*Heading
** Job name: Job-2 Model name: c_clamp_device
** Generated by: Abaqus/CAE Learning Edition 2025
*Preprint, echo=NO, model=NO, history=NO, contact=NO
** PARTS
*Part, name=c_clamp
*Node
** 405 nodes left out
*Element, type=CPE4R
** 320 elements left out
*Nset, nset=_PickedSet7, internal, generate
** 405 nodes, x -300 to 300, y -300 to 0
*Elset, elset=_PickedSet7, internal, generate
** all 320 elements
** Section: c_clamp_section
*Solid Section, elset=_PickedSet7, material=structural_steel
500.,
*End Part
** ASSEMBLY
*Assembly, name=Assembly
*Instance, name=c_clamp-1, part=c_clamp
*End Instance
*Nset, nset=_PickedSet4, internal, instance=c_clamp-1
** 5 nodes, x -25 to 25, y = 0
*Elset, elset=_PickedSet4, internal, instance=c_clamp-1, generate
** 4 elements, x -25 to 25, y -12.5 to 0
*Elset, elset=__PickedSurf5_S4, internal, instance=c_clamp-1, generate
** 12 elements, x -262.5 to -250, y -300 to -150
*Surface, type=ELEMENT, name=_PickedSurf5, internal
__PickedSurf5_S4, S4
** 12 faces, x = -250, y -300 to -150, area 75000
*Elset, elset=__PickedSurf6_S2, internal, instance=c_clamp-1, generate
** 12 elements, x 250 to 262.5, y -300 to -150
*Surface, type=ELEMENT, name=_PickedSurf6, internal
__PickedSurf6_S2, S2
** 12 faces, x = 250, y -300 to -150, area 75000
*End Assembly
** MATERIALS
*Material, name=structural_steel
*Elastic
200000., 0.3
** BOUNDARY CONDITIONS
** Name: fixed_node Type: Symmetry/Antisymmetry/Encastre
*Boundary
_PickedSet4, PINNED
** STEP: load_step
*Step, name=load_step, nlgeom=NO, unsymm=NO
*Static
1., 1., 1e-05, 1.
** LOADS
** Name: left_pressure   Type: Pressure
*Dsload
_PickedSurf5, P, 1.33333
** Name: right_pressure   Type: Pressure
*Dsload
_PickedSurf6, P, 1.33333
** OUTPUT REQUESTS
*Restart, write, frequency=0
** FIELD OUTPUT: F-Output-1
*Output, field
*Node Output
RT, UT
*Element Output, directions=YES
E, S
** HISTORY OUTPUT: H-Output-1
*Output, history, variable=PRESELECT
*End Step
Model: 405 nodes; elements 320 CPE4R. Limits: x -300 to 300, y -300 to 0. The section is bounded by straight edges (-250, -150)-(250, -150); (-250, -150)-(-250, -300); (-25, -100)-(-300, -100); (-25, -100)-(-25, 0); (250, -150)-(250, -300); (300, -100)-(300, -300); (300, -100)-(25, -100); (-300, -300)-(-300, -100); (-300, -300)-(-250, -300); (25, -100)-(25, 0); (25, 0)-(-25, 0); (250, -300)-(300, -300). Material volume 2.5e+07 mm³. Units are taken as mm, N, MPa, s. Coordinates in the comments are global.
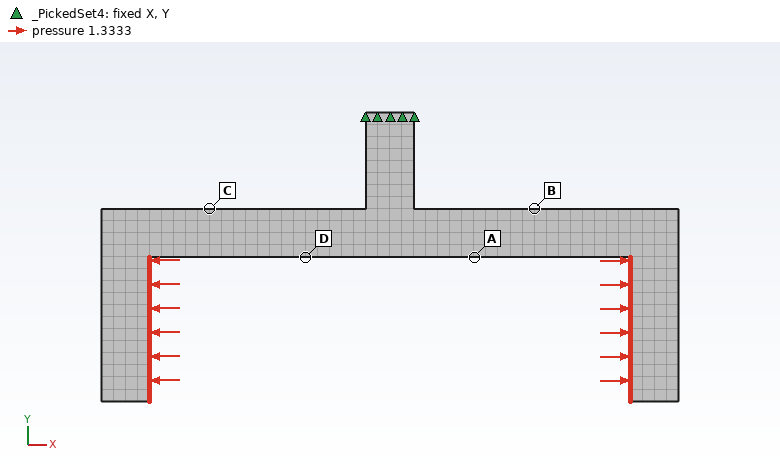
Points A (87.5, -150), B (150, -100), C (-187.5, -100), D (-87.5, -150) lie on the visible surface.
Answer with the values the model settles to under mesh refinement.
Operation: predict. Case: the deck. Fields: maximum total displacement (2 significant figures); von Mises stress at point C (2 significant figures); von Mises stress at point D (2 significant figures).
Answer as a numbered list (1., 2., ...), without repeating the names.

1. 0.60 mm
2. 39 MPa
3. 46 MPa
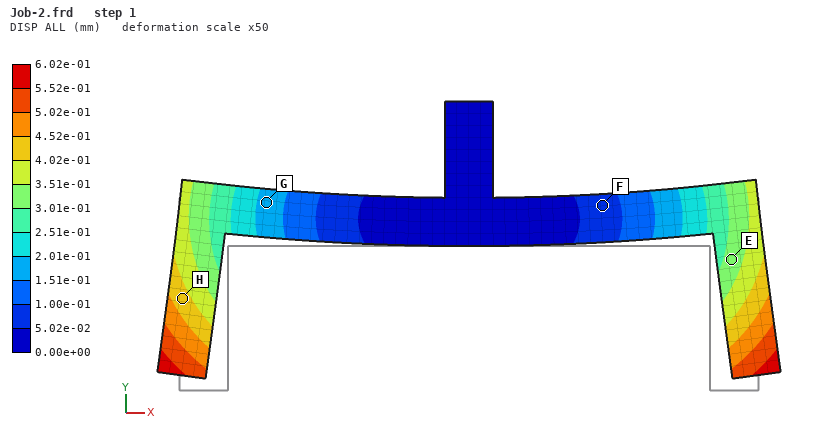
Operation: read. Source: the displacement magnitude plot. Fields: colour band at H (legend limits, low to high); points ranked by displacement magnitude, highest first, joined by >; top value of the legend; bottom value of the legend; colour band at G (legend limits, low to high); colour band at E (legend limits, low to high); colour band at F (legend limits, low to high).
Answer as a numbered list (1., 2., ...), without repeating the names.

1. 4.02e-01 to 4.52e-01 mm
2. H > E > G > F
3. 6.02e-01 mm
4. 0.00e+00 mm
5. 1.51e-01 to 2.01e-01 mm
6. 3.01e-01 to 3.51e-01 mm
7. 5.02e-02 to 1.00e-01 mm
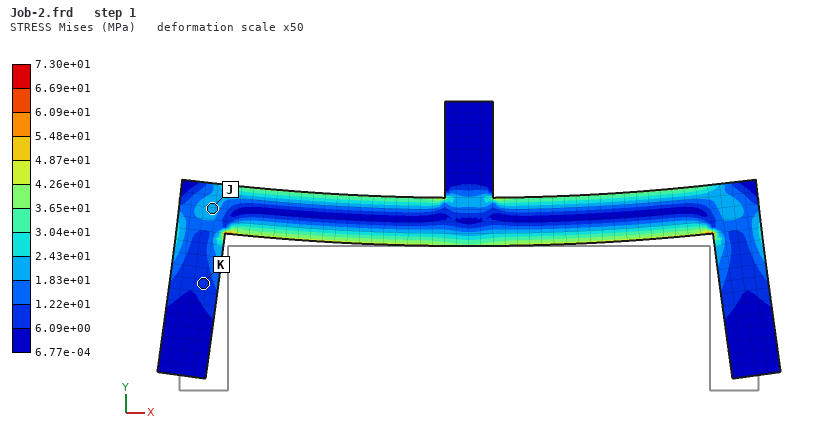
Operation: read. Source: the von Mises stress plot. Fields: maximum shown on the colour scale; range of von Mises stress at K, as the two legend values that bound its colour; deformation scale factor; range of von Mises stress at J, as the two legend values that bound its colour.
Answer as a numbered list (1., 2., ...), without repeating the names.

1. 7.30e+01 MPa
2. 6.09e+00 to 1.22e+01 MPa
3. 50
4. 1.83e+01 to 2.43e+01 MPa
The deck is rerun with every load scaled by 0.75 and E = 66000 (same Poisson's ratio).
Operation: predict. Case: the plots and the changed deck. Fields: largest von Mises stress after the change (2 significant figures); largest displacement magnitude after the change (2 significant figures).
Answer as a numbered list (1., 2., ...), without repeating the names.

1. 55 MPa
2. 1.4 mm
